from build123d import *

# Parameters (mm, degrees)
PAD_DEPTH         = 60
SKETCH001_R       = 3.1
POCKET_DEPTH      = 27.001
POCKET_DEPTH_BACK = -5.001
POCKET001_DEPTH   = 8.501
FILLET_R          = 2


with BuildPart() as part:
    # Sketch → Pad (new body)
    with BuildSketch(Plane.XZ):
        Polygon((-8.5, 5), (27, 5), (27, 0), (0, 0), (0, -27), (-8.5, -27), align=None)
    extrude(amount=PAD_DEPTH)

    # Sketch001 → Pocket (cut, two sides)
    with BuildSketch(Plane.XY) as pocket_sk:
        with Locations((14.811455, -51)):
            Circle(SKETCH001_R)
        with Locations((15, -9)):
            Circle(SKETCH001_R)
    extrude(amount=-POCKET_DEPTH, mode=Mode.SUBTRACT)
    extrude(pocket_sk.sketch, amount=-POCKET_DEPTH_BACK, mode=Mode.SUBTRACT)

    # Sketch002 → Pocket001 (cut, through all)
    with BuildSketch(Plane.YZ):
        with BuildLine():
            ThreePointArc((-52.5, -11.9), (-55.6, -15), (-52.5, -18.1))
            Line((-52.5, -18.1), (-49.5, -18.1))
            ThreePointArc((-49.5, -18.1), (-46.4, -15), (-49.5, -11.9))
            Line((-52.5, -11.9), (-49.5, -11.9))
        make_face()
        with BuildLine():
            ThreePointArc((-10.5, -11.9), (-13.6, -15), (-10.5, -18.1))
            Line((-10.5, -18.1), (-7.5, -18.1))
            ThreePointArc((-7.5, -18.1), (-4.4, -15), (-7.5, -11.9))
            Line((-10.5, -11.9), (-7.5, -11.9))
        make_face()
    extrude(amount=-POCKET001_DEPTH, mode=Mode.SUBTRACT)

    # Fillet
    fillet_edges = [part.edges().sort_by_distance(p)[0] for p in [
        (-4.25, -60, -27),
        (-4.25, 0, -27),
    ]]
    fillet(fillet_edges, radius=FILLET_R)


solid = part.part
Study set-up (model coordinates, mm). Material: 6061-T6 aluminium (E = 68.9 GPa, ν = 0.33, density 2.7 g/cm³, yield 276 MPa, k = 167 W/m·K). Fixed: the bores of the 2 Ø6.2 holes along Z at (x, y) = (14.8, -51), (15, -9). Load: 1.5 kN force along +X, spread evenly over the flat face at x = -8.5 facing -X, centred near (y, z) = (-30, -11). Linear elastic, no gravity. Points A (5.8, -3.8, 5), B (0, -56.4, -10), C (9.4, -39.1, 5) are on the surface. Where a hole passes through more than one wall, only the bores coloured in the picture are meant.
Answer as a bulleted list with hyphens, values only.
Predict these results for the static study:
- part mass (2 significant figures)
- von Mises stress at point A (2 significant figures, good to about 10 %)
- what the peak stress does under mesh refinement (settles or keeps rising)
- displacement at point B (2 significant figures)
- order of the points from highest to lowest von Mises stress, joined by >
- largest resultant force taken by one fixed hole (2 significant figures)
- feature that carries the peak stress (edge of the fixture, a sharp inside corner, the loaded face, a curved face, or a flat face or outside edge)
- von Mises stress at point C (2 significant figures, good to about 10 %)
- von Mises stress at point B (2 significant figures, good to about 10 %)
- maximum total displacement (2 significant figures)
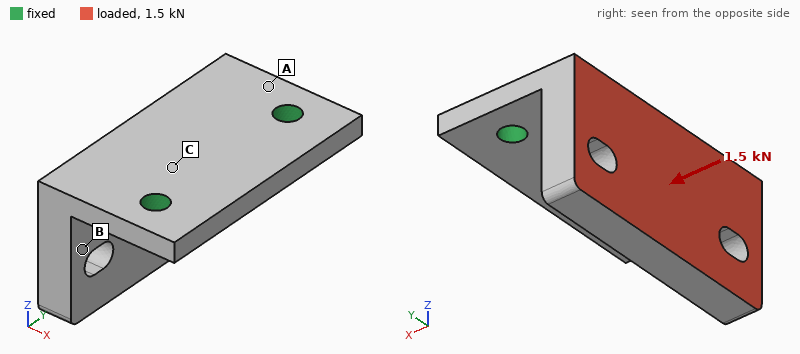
- 63 g
- 76 MPa
- keeps rising
- 0.11 mm
- A > C > B
- 770 N
- edge of the fixture
- 51 MPa
- 11 MPa
- 0.27 mm
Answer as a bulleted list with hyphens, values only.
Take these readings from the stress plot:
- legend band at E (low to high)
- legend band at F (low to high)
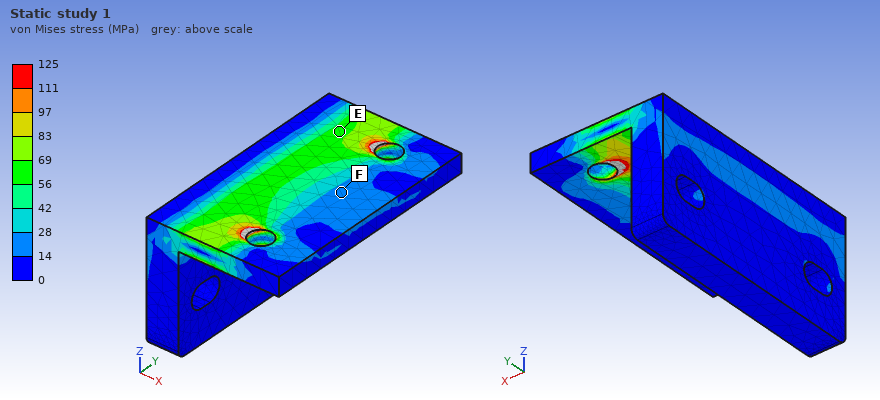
- 56 to 69 MPa
- 14 to 28 MPa
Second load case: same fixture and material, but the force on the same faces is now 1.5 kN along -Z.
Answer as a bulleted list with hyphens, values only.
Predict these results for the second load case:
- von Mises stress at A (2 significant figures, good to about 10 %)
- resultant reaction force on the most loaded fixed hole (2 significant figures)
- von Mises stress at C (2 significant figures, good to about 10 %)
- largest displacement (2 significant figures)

- 93 MPa
- 750 N
- 64 MPa
- 0.30 mm
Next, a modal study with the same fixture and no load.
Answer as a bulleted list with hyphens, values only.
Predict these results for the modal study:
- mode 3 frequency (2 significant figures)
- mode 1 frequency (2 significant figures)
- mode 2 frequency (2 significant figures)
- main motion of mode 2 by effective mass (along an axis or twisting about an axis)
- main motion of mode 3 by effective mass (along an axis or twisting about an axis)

- 7000 Hz
- 2000 Hz
- 4600 Hz
- along Y
- along Z
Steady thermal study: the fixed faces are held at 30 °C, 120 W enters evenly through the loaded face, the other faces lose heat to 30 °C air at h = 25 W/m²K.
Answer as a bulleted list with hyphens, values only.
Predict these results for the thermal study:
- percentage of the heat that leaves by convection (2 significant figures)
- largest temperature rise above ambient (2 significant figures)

- 5.4 %
- 66 K
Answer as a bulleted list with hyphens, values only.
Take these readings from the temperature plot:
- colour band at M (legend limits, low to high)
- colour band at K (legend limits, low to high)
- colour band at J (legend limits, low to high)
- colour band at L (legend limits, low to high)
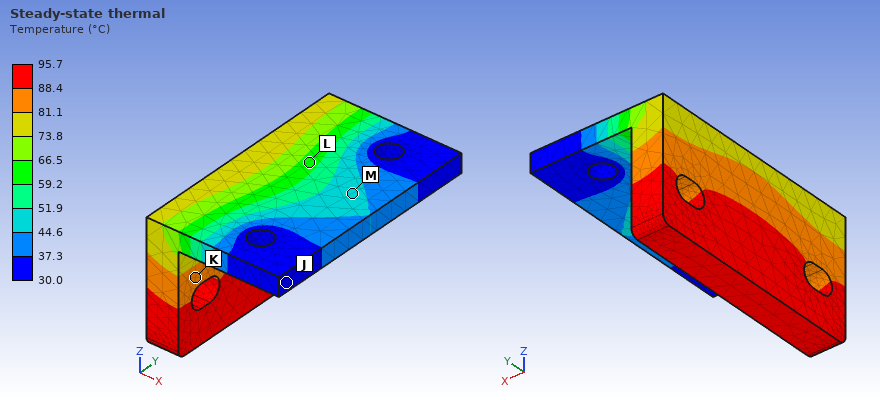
- 44.6 to 51.9 °C
- 81.1 to 88.4 °C
- 30.0 to 37.3 °C
- 59.2 to 66.5 °C
